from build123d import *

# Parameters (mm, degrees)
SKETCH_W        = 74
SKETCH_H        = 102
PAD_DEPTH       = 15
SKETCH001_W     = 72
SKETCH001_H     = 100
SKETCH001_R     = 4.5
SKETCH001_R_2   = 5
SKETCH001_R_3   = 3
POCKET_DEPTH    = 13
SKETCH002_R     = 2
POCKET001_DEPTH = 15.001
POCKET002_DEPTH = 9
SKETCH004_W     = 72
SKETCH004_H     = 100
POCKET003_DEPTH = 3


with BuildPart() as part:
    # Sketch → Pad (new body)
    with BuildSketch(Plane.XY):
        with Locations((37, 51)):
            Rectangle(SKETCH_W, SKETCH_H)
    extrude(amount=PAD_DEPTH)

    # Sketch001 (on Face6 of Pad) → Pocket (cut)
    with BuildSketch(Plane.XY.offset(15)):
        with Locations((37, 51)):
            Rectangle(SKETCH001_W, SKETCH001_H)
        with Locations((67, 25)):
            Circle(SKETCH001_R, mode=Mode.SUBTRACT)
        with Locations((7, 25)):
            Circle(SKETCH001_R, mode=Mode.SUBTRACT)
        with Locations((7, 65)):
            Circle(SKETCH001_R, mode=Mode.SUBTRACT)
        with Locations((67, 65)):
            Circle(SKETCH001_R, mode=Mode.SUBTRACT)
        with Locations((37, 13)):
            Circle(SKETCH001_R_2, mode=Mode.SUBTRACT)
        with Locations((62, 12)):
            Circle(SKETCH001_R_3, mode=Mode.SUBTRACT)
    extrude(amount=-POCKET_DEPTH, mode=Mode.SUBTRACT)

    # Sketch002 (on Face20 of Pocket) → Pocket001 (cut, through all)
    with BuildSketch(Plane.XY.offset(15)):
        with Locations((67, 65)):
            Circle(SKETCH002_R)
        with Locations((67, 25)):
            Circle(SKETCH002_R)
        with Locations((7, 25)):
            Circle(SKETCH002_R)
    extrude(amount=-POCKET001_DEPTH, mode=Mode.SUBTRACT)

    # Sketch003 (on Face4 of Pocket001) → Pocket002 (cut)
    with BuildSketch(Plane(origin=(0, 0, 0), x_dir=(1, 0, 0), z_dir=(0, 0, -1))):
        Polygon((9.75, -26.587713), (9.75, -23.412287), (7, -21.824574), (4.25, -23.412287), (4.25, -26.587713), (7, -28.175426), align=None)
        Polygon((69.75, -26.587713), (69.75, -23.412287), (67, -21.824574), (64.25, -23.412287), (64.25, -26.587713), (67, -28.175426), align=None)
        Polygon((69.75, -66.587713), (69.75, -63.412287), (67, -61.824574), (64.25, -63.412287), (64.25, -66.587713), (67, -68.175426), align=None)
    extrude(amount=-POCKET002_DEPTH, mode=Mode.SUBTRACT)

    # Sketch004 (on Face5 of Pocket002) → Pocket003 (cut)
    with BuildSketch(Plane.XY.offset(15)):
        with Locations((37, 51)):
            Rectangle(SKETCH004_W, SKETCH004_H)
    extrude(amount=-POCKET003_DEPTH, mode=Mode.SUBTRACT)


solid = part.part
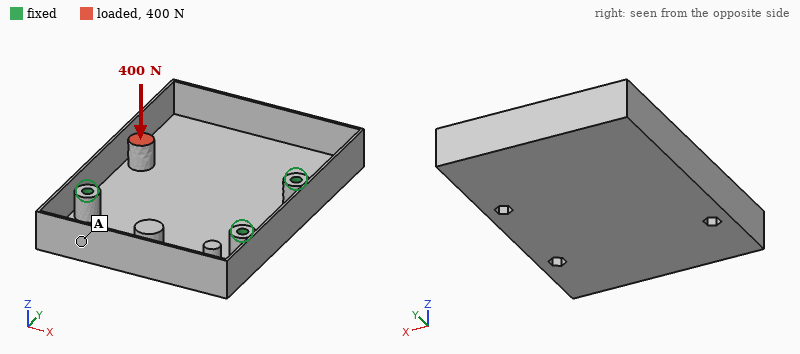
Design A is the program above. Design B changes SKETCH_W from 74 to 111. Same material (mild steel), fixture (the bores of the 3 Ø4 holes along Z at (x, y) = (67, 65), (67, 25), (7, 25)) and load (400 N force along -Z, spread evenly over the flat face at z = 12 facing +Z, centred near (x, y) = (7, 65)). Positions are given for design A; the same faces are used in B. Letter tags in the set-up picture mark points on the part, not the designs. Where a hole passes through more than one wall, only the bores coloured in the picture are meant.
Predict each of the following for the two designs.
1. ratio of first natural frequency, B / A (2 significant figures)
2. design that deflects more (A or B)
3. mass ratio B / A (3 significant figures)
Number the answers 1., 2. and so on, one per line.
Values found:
1. 1.1
2. A
3. 3.53
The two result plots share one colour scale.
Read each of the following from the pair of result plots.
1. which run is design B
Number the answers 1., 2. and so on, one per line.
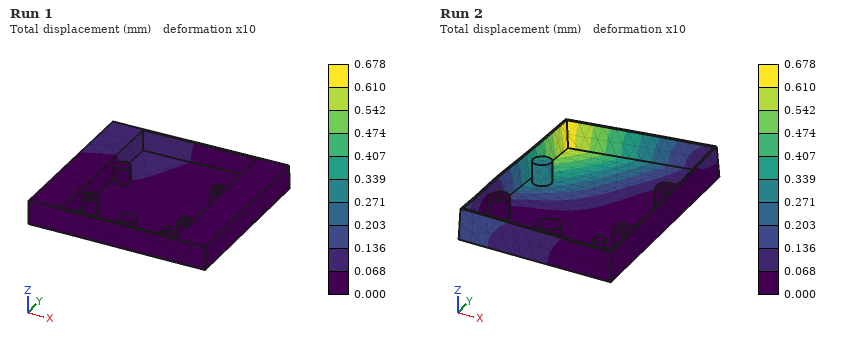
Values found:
1. Run 1
